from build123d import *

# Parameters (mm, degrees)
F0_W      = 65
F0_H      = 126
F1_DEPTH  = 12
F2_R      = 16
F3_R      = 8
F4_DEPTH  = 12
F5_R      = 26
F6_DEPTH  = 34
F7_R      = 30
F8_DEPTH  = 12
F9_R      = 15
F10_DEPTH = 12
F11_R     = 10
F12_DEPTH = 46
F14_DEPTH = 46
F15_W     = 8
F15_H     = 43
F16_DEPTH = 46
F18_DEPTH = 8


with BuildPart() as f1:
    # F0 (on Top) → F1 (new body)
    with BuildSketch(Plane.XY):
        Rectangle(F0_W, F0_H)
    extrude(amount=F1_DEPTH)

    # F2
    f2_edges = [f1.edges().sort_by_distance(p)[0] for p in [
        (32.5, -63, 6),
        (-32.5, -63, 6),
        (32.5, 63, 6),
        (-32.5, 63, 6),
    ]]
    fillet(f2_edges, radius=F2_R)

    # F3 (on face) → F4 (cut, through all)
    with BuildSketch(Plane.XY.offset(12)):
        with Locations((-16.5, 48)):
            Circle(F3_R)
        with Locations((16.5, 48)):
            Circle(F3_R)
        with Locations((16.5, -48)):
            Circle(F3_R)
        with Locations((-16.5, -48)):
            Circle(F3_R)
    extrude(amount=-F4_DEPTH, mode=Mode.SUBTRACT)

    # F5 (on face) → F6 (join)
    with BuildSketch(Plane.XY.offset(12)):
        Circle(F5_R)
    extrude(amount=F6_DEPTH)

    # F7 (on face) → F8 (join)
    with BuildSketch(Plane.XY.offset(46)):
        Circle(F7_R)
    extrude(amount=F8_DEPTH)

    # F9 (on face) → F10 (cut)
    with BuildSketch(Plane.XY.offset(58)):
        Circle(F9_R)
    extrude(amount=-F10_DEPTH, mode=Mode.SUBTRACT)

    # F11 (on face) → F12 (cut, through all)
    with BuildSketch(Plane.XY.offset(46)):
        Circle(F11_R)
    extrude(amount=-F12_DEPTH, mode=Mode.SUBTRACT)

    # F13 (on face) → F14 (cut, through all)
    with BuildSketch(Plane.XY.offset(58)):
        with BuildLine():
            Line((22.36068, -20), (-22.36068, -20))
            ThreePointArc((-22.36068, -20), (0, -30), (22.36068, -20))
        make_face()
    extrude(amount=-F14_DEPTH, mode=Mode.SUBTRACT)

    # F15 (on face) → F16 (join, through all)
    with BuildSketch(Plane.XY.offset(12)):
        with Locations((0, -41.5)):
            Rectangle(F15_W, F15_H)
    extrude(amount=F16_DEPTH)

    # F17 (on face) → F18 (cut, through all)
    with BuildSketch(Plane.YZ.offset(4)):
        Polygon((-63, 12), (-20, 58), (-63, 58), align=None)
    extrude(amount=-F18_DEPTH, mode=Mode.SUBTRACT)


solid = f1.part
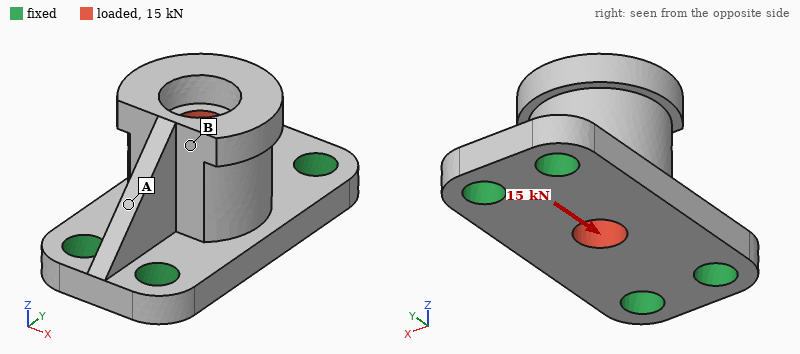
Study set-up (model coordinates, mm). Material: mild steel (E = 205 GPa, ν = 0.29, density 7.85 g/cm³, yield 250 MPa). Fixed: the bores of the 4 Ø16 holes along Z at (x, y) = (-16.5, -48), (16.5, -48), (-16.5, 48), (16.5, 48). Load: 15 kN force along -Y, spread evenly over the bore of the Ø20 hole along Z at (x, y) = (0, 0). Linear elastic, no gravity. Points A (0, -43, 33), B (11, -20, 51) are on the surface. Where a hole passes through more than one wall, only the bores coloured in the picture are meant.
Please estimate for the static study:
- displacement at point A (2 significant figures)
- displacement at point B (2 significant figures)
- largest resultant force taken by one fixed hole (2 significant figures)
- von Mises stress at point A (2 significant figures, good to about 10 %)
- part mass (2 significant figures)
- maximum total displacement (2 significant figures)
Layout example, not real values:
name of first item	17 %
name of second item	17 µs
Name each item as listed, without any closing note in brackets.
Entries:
displacement at point A	3.6 µm
displacement at point B	6.1 µm
largest resultant force taken by one fixed hole	4.5 kN
von Mises stress at point A	14 MPa
part mass	1.3 kg
maximum total displacement	8.4 µm
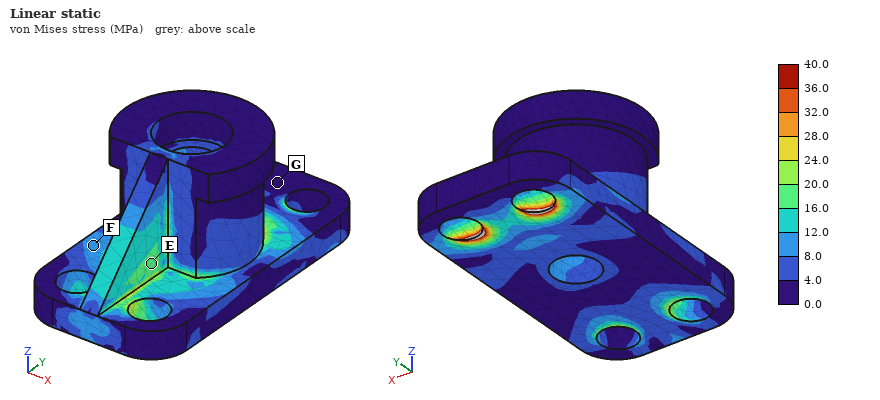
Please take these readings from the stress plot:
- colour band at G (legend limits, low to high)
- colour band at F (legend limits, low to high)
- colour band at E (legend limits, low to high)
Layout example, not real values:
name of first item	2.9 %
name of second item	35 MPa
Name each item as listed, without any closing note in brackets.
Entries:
colour band at G	0.0 to 4.0 MPa
colour band at F	8.0 to 12.0 MPa
colour band at E	16.0 to 20.0 MPa
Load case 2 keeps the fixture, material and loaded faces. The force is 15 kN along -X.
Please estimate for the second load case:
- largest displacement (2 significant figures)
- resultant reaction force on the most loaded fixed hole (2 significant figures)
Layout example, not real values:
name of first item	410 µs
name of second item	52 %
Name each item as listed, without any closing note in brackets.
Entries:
largest displacement	36 µm
resultant reaction force on the most loaded fixed hole	6.2 kN
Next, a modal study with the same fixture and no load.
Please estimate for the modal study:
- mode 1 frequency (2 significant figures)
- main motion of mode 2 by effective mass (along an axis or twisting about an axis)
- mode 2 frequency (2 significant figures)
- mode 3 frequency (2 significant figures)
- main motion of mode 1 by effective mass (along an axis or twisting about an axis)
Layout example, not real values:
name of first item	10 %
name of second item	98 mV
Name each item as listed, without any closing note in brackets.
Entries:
mode 1 frequency	3500 Hz
main motion of mode 2 by effective mass	along Z
mode 2 frequency	6000 Hz
mode 3 frequency	8100 Hz
main motion of mode 1 by effective mass	along X
